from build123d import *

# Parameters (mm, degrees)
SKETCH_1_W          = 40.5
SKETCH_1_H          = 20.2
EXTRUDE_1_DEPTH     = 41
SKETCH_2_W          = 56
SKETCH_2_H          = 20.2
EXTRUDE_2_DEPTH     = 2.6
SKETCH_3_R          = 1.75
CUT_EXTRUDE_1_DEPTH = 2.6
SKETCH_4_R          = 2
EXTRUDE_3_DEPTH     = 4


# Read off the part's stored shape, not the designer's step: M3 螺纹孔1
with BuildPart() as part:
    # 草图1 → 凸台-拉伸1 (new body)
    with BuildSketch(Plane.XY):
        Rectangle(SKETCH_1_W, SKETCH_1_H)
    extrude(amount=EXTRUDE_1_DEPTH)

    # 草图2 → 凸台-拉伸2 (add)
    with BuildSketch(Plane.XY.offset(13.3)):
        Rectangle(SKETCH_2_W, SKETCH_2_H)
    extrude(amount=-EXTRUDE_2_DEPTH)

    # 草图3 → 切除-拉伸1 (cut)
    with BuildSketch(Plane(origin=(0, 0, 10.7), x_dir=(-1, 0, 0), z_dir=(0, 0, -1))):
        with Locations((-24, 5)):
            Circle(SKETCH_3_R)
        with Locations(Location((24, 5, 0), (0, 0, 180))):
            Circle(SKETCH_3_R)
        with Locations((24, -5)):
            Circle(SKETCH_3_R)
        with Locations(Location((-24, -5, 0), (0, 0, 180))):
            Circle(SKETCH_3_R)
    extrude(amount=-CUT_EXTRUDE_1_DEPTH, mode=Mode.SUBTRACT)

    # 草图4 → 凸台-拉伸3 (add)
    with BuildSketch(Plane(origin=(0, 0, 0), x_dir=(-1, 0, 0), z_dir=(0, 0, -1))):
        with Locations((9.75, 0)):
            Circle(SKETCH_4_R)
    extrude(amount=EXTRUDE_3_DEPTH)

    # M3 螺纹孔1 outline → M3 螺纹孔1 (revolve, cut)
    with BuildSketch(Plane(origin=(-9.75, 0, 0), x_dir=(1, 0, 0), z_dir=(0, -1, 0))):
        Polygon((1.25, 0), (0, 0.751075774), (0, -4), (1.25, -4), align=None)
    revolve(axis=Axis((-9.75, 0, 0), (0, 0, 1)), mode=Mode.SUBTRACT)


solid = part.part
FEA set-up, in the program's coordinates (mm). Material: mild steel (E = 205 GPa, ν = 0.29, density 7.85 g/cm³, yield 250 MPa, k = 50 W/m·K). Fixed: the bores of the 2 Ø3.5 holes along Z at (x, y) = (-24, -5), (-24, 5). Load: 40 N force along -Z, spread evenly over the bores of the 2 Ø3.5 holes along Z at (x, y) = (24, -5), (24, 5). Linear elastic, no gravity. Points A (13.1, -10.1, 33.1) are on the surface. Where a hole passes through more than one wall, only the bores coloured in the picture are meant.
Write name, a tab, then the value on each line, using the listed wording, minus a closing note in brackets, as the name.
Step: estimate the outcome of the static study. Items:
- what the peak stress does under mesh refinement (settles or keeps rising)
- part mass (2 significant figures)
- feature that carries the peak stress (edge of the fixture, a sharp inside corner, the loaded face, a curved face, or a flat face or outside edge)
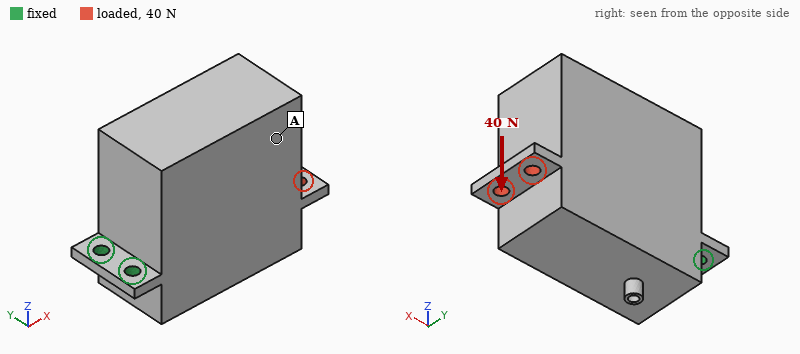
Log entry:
what the peak stress does under mesh refinement	keeps rising
part mass	270 g
feature that carries the peak stress	edge of the fixture
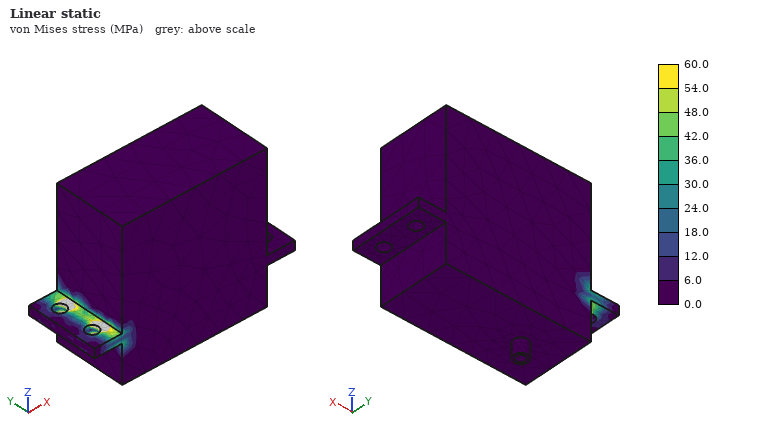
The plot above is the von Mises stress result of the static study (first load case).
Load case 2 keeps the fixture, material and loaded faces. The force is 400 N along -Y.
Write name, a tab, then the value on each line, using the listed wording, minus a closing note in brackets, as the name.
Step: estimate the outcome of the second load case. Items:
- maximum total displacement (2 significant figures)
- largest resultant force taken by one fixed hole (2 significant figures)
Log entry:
maximum total displacement	24 µm
largest resultant force taken by one fixed hole	1.6 kN
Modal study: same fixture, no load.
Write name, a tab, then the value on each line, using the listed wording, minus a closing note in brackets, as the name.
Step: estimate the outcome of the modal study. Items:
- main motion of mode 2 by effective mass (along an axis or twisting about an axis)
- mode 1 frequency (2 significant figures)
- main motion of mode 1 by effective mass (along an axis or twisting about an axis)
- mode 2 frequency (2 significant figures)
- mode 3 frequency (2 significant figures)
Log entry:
main motion of mode 2 by effective mass	along Y
mode 1 frequency	440 Hz
main motion of mode 1 by effective mass	along Z
mode 2 frequency	2100 Hz
mode 3 frequency	3400 Hz
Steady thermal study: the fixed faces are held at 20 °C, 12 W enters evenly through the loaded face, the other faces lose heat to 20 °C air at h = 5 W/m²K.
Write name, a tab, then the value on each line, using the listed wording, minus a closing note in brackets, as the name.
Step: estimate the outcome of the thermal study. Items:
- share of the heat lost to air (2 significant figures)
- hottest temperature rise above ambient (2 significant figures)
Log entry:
share of the heat lost to air	8.4 %
hottest temperature rise above ambient	70 K
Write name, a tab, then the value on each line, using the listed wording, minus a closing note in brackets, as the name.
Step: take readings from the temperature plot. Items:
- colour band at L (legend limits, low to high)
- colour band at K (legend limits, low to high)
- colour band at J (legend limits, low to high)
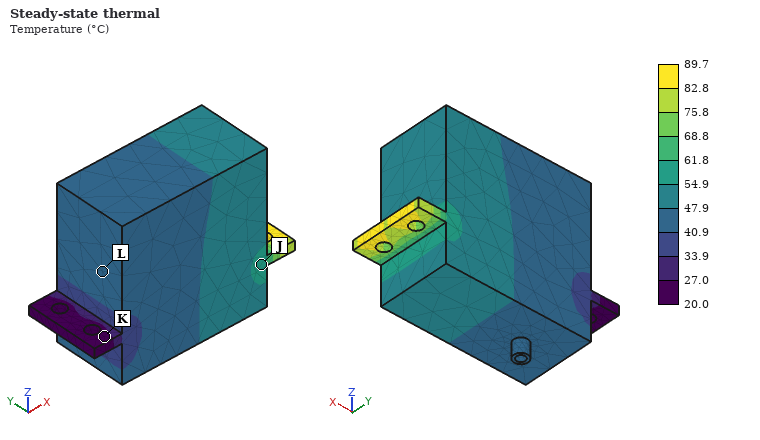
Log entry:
colour band at L	40.9 to 47.9 °C
colour band at K	20.0 to 27.0 °C
colour band at J	54.9 to 61.8 °C
